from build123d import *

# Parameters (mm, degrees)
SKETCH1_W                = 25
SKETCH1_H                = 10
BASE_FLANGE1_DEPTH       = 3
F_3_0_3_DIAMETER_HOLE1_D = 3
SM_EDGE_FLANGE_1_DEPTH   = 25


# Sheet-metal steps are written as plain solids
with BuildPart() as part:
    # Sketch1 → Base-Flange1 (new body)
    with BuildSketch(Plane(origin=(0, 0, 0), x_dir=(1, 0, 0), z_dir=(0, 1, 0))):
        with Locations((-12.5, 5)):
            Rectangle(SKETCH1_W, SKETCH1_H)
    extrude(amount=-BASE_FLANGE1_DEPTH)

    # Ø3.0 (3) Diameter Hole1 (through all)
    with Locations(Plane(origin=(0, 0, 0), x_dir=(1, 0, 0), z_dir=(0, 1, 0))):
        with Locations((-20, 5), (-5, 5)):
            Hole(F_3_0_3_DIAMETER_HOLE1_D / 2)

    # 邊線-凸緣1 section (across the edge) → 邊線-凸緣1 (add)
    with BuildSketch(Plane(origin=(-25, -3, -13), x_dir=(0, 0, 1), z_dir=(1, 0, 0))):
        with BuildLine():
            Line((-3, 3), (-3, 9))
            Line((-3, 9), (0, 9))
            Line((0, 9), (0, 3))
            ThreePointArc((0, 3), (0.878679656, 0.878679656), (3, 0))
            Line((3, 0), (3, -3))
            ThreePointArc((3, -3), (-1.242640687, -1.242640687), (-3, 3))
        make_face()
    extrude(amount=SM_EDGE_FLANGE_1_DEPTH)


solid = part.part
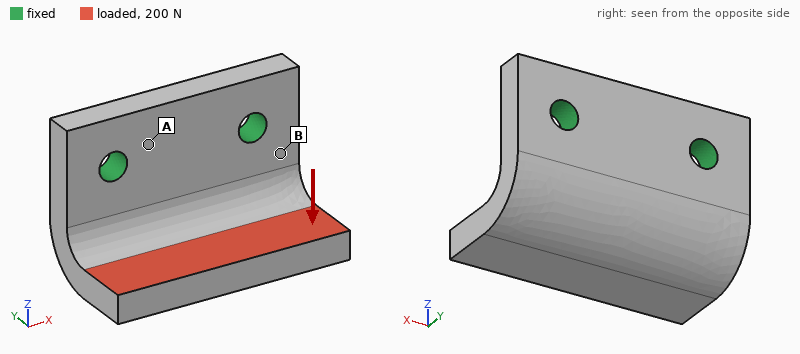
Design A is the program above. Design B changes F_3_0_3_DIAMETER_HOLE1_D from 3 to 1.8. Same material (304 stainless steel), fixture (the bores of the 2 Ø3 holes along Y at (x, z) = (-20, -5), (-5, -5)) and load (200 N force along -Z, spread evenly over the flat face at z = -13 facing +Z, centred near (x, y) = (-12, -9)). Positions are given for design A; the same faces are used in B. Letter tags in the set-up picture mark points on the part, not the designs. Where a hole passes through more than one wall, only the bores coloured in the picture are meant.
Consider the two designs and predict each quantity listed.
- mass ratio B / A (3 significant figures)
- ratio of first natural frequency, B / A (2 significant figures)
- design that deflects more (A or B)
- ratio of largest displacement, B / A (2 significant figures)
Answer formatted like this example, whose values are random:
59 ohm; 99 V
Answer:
1.02; 0.89; B; 1.2
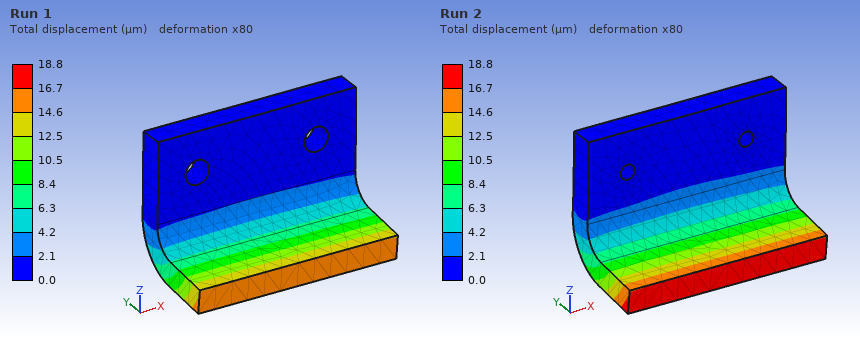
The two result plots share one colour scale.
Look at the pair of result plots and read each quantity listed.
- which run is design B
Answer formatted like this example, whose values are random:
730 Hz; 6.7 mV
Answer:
Run 2
